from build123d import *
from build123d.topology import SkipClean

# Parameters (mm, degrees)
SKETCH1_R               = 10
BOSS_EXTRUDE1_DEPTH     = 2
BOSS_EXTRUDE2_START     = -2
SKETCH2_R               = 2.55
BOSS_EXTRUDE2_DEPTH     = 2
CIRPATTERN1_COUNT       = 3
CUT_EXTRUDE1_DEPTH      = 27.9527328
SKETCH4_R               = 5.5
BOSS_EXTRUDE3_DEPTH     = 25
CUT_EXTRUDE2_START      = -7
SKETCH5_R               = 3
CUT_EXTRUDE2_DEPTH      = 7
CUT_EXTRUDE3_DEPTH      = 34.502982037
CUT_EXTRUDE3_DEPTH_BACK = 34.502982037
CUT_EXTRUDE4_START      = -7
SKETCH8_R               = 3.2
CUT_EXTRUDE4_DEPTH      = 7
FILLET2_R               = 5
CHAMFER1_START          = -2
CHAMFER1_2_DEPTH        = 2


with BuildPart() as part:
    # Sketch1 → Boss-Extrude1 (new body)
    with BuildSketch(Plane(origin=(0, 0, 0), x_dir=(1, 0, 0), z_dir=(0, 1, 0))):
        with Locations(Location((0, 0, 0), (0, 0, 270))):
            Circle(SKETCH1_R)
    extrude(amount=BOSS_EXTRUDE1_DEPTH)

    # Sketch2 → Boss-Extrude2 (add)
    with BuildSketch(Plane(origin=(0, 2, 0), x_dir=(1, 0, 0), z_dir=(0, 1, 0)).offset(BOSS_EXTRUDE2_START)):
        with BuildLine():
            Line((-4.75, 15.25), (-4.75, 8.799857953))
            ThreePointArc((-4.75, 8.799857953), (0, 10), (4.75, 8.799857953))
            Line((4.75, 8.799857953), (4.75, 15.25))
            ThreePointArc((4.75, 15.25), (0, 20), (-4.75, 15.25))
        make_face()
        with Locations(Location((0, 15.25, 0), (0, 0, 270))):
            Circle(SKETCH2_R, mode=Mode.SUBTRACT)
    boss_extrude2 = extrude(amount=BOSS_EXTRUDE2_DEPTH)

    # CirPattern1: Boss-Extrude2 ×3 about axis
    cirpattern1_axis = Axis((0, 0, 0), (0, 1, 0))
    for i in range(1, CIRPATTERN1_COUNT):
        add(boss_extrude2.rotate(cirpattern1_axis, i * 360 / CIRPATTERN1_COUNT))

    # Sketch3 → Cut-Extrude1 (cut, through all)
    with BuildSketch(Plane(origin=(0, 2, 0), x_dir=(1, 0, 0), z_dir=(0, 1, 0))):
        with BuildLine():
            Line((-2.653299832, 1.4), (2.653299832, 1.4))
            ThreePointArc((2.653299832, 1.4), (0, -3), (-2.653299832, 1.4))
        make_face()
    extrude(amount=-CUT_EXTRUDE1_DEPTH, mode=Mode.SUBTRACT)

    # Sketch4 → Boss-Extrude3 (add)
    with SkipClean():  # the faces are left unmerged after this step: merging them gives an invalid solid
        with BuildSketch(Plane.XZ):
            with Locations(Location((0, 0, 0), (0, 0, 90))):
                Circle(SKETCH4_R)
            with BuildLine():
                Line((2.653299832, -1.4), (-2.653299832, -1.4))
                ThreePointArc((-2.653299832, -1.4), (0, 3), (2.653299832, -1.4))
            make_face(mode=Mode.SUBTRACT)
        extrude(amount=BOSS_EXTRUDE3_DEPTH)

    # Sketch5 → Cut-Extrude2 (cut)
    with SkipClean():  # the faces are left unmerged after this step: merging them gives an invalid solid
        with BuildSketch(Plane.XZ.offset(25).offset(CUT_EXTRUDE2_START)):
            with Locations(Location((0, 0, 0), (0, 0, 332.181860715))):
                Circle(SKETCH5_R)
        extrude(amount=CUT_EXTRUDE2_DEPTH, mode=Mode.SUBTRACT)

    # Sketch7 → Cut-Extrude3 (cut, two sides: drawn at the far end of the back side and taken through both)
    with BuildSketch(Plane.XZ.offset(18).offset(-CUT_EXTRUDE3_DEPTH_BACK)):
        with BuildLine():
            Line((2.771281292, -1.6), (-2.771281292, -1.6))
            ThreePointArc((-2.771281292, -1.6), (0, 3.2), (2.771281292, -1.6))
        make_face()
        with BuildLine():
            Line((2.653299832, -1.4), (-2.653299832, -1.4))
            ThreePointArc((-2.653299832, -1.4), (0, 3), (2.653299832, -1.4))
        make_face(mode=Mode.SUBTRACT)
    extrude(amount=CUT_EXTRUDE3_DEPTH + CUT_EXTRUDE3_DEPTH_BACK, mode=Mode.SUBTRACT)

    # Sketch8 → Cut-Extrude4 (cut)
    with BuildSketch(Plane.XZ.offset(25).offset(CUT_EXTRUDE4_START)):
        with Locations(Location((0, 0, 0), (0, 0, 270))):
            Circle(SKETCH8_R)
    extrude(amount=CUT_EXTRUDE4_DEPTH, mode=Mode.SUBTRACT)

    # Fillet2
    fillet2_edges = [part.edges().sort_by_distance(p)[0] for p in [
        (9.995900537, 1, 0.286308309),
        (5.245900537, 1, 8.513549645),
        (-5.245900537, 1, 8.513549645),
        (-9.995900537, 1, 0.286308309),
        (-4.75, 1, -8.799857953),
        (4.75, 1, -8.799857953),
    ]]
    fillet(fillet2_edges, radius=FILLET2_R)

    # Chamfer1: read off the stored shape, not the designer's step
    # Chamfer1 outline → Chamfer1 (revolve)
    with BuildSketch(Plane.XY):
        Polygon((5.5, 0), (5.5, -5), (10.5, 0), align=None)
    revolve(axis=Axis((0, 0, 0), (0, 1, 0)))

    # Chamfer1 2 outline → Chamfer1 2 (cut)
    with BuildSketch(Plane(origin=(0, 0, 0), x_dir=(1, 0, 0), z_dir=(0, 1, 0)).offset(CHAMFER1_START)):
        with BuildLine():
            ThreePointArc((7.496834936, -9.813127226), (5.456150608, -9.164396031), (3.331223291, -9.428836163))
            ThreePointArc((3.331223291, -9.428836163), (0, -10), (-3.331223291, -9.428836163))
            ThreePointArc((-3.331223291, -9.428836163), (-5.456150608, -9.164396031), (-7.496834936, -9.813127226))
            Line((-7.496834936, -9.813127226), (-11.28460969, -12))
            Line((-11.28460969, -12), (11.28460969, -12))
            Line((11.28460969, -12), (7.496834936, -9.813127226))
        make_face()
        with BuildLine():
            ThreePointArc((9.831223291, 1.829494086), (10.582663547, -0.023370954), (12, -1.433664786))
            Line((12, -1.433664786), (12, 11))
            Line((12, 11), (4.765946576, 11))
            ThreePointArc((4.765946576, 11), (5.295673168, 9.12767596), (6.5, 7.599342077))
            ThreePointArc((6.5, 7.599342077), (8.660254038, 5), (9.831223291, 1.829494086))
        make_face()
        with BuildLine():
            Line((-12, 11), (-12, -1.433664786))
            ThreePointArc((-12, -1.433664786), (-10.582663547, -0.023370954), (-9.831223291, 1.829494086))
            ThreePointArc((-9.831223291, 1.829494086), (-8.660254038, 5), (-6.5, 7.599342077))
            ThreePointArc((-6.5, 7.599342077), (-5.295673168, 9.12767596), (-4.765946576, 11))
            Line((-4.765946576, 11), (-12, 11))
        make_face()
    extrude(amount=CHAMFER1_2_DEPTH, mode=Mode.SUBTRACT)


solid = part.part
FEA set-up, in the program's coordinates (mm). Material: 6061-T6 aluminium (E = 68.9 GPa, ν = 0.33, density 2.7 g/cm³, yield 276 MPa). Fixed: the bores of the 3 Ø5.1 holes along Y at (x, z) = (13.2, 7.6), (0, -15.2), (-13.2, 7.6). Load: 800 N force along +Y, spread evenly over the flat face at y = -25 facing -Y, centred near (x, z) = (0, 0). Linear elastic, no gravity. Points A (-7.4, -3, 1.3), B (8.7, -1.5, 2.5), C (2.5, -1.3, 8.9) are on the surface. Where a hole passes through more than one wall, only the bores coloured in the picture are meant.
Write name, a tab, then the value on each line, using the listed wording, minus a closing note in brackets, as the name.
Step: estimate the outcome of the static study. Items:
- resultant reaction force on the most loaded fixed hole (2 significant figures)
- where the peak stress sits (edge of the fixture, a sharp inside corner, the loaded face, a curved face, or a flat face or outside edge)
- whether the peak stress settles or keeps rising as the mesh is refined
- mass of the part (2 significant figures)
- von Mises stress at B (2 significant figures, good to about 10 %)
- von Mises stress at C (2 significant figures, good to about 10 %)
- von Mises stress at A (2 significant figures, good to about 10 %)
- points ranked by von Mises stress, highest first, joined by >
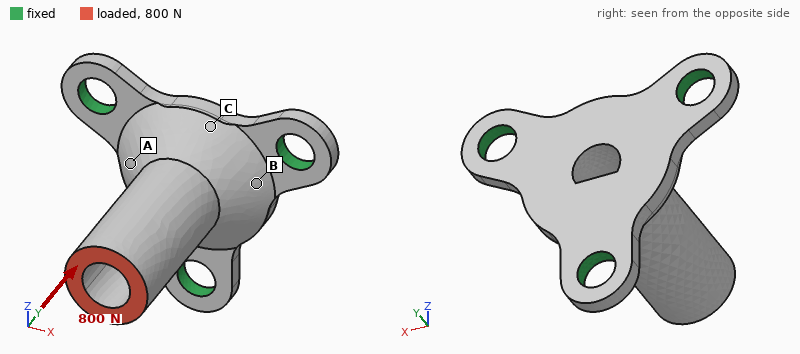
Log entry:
resultant reaction force on the most loaded fixed hole	360 N
where the peak stress sits	edge of the fixture
whether the peak stress settles or keeps rising as the mesh is refined	keeps rising
mass of the part	8.8 g
von Mises stress at B	38 MPa
von Mises stress at C	12 MPa
von Mises stress at A	25 MPa
points ranked by von Mises stress, highest first, joined by >	B > A > C
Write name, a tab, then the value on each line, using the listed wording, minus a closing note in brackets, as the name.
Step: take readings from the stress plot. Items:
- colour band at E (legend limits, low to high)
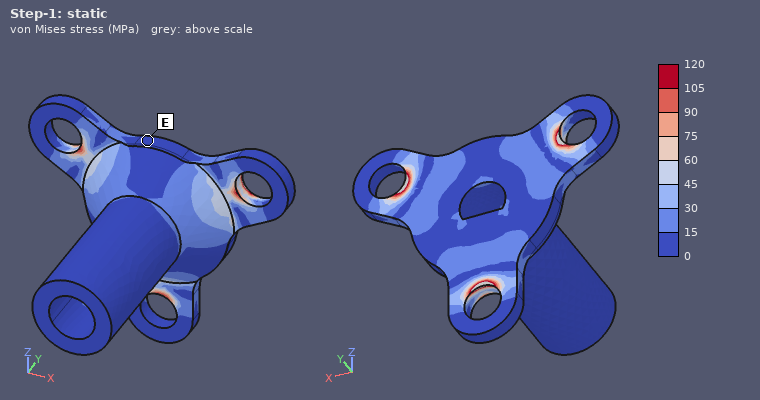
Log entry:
colour band at E	0 to 15 MPa
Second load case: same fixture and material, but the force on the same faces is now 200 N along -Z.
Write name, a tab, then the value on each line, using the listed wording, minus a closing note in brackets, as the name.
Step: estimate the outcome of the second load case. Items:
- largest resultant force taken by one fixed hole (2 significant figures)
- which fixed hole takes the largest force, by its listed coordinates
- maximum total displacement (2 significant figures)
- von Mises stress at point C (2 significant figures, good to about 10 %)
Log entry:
largest resultant force taken by one fixed hole	340 N
which fixed hole takes the largest force, by its listed coordinates	(0, -15.2)
maximum total displacement	48 µm
von Mises stress at point C	12 MPa
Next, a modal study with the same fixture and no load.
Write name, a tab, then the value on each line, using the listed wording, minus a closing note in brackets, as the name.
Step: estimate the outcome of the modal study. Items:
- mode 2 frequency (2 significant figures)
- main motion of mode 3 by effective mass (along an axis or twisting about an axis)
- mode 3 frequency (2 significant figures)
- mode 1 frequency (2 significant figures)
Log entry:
mode 2 frequency	9000 Hz
main motion of mode 3 by effective mass	along Y
mode 3 frequency	16 kHz
mode 1 frequency	9000 Hz
